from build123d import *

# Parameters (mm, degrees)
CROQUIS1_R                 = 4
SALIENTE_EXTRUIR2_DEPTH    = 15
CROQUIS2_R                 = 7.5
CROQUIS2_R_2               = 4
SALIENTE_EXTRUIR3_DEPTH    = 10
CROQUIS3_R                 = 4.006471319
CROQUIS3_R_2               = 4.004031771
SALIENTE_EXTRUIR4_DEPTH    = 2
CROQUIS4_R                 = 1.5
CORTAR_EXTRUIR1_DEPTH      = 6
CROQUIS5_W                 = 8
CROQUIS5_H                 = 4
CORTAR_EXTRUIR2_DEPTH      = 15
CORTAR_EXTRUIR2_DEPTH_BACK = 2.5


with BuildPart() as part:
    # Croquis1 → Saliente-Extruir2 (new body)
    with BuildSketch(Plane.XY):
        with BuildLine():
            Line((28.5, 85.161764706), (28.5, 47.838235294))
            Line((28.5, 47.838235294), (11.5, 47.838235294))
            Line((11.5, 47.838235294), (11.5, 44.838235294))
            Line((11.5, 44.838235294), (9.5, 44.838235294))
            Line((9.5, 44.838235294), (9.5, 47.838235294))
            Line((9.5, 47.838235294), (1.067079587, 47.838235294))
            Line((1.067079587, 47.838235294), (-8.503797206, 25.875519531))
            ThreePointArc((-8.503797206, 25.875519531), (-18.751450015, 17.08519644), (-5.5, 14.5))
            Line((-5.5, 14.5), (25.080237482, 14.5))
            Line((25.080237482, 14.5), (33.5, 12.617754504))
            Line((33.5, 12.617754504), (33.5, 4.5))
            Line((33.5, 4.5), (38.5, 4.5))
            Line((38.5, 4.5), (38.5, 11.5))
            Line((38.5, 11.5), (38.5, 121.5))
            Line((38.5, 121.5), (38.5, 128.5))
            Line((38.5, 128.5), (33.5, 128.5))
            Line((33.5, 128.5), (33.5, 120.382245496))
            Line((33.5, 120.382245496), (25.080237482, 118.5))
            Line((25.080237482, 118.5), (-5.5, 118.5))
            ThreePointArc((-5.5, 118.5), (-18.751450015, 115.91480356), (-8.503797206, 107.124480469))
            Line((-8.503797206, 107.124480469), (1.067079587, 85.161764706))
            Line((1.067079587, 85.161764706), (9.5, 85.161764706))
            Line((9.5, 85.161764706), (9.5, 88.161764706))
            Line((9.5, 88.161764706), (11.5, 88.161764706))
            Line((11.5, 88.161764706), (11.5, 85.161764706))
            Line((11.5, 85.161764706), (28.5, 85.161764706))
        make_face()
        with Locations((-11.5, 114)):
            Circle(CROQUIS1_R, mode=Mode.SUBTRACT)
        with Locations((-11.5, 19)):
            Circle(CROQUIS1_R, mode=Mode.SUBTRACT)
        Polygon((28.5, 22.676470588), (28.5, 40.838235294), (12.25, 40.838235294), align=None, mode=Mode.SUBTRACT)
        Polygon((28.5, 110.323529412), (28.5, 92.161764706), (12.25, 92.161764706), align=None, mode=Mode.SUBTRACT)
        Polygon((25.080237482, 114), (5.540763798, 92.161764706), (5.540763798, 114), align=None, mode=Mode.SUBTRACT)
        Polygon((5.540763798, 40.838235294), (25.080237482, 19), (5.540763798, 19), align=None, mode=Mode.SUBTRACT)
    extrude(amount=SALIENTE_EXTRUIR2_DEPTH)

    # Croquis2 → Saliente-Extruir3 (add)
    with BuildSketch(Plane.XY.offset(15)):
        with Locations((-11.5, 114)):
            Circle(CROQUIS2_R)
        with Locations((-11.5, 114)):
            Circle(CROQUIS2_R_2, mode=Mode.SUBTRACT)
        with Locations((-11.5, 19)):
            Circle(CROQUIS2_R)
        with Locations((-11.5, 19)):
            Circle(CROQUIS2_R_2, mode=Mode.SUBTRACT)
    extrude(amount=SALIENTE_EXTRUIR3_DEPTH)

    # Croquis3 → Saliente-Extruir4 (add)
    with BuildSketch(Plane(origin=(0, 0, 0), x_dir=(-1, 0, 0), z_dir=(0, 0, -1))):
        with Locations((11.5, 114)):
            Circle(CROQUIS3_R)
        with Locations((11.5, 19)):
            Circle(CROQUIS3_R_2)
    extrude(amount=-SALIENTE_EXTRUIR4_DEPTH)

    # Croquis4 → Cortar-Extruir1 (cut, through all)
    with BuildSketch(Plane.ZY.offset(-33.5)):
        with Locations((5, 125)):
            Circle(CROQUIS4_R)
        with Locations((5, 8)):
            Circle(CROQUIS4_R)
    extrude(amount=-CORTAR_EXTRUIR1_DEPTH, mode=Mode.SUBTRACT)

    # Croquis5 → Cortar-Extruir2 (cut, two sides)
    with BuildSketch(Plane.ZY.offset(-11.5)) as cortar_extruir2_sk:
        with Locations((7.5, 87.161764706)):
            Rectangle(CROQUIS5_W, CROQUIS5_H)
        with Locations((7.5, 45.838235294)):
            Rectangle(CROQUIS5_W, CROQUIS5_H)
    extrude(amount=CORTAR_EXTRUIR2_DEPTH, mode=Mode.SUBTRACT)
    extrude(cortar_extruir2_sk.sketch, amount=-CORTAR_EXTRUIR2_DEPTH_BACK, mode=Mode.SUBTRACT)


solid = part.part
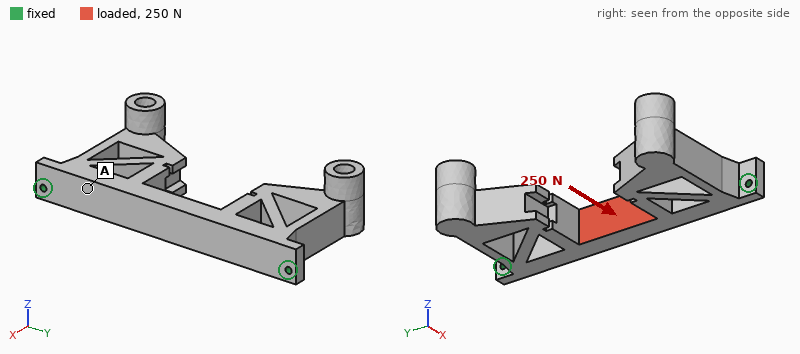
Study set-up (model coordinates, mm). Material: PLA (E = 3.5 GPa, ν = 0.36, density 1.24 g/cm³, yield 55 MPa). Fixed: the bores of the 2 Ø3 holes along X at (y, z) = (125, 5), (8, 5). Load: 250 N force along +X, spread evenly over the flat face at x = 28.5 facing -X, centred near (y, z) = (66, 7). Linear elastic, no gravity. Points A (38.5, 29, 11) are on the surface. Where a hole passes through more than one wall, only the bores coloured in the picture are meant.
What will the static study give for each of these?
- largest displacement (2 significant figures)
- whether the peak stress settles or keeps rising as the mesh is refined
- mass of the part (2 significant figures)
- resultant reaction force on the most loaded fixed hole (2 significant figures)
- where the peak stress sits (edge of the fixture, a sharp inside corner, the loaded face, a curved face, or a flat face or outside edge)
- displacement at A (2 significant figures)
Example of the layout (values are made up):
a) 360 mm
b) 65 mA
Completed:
a) 1.0 mm
b) keeps rising
c) 55 g
d) 310 N
e) edge of the fixture
f) 0.38 mm
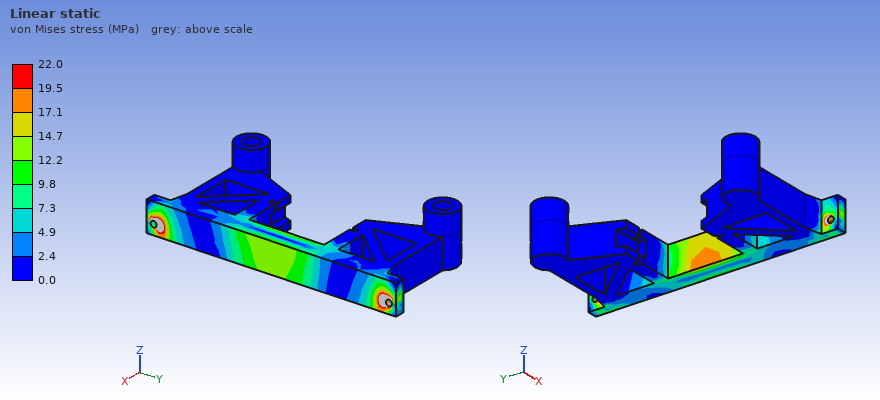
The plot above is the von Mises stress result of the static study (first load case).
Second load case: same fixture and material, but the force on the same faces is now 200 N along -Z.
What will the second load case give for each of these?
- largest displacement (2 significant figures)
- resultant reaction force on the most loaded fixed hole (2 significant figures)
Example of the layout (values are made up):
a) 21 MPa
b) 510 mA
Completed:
a) 0.63 mm
b) 150 N
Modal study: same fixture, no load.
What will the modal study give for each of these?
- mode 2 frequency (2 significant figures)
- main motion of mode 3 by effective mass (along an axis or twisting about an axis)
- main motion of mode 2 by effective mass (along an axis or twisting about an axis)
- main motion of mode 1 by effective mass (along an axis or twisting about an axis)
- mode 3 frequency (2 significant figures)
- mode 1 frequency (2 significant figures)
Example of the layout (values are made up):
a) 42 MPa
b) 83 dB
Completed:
a) 460 Hz
b) twisting about X
c) along X
d) along Z
e) 530 Hz
f) 320 Hz
